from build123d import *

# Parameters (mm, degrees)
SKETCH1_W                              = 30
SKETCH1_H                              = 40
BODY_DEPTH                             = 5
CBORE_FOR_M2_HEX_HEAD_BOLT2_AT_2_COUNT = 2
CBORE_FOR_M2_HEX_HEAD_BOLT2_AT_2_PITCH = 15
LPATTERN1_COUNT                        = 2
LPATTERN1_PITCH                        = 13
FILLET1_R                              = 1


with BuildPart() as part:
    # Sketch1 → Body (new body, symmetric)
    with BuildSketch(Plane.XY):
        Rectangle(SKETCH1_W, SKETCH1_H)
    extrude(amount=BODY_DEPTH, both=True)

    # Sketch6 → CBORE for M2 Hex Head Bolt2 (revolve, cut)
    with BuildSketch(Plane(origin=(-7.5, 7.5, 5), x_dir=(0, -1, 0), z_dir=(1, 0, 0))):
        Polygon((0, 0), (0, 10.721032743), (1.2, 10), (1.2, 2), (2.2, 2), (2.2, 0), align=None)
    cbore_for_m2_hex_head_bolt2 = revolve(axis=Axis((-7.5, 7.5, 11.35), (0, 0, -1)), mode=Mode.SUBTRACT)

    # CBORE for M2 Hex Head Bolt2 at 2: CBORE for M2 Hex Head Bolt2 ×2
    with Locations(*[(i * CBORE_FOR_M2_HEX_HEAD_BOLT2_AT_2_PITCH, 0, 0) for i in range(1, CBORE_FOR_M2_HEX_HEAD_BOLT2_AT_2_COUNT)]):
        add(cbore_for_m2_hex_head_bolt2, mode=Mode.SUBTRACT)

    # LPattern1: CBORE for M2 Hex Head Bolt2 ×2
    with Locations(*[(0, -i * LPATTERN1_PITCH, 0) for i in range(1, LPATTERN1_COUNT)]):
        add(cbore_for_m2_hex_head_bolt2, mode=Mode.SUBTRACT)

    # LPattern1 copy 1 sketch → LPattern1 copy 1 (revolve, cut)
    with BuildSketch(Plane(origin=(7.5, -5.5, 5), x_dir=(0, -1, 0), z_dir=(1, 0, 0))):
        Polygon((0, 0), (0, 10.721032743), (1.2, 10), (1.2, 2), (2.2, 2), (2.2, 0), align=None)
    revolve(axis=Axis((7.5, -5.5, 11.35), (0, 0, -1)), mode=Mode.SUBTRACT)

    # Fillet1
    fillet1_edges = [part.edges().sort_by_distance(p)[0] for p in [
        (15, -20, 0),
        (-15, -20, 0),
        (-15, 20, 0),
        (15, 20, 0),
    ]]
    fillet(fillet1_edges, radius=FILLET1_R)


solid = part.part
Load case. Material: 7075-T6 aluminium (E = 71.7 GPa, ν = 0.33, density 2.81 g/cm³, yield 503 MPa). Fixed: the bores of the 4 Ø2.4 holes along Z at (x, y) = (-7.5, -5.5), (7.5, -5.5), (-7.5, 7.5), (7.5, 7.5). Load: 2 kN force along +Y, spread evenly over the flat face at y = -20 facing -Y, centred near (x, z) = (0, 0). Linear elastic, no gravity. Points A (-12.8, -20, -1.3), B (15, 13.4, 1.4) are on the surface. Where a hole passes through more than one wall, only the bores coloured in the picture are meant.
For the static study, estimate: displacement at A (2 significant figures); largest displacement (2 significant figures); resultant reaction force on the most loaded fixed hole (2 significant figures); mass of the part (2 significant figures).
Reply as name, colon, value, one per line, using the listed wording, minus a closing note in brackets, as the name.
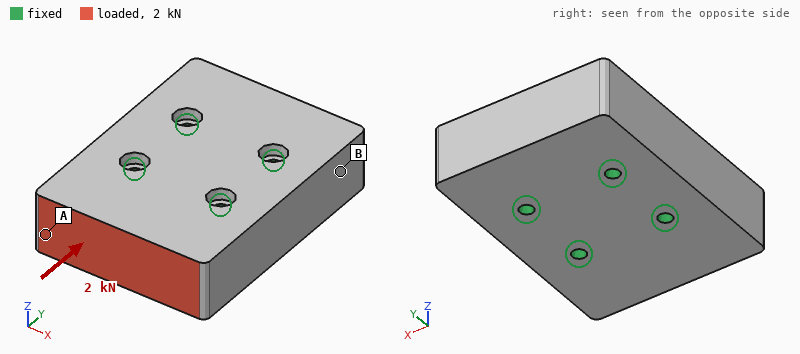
displacement at A: 1.7 µm
largest displacement: 2.2 µm
resultant reaction force on the most loaded fixed hole: 780 N
mass of the part: 33 g
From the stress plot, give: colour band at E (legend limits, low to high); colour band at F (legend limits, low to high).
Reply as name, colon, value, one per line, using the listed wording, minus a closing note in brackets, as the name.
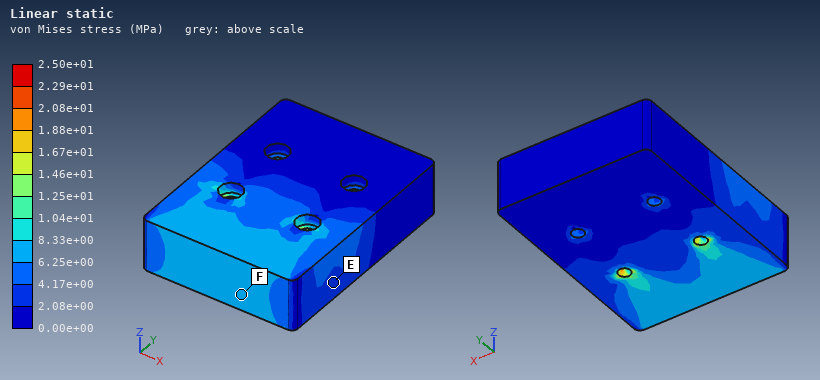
colour band at E: 2.08e+00 to 4.17e+00 MPa
colour band at F: 6.25e+00 to 8.33e+00 MPa
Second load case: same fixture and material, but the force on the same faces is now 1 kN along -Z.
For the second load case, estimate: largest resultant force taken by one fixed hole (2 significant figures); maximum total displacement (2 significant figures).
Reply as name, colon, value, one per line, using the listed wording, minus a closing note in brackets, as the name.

largest resultant force taken by one fixed hole: 730 N
maximum total displacement: 13 µm
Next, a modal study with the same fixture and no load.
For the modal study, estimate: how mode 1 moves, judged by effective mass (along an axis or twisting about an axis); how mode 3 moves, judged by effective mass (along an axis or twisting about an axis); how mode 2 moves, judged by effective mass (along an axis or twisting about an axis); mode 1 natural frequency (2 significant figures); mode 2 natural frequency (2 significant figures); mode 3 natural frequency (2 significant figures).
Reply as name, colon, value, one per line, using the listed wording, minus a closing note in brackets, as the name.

how mode 1 moves, judged by effective mass: along Z
how mode 3 moves, judged by effective mass: twisting about Y
how mode 2 moves, judged by effective mass: along Z
mode 1 natural frequency: 23 kHz
mode 2 natural frequency: 28 kHz
mode 3 natural frequency: 31 kHz
